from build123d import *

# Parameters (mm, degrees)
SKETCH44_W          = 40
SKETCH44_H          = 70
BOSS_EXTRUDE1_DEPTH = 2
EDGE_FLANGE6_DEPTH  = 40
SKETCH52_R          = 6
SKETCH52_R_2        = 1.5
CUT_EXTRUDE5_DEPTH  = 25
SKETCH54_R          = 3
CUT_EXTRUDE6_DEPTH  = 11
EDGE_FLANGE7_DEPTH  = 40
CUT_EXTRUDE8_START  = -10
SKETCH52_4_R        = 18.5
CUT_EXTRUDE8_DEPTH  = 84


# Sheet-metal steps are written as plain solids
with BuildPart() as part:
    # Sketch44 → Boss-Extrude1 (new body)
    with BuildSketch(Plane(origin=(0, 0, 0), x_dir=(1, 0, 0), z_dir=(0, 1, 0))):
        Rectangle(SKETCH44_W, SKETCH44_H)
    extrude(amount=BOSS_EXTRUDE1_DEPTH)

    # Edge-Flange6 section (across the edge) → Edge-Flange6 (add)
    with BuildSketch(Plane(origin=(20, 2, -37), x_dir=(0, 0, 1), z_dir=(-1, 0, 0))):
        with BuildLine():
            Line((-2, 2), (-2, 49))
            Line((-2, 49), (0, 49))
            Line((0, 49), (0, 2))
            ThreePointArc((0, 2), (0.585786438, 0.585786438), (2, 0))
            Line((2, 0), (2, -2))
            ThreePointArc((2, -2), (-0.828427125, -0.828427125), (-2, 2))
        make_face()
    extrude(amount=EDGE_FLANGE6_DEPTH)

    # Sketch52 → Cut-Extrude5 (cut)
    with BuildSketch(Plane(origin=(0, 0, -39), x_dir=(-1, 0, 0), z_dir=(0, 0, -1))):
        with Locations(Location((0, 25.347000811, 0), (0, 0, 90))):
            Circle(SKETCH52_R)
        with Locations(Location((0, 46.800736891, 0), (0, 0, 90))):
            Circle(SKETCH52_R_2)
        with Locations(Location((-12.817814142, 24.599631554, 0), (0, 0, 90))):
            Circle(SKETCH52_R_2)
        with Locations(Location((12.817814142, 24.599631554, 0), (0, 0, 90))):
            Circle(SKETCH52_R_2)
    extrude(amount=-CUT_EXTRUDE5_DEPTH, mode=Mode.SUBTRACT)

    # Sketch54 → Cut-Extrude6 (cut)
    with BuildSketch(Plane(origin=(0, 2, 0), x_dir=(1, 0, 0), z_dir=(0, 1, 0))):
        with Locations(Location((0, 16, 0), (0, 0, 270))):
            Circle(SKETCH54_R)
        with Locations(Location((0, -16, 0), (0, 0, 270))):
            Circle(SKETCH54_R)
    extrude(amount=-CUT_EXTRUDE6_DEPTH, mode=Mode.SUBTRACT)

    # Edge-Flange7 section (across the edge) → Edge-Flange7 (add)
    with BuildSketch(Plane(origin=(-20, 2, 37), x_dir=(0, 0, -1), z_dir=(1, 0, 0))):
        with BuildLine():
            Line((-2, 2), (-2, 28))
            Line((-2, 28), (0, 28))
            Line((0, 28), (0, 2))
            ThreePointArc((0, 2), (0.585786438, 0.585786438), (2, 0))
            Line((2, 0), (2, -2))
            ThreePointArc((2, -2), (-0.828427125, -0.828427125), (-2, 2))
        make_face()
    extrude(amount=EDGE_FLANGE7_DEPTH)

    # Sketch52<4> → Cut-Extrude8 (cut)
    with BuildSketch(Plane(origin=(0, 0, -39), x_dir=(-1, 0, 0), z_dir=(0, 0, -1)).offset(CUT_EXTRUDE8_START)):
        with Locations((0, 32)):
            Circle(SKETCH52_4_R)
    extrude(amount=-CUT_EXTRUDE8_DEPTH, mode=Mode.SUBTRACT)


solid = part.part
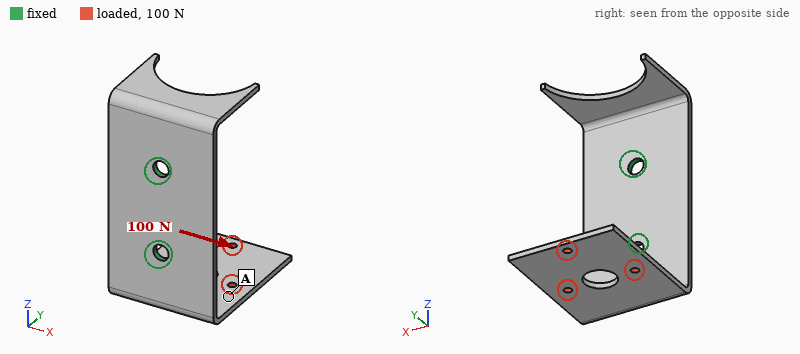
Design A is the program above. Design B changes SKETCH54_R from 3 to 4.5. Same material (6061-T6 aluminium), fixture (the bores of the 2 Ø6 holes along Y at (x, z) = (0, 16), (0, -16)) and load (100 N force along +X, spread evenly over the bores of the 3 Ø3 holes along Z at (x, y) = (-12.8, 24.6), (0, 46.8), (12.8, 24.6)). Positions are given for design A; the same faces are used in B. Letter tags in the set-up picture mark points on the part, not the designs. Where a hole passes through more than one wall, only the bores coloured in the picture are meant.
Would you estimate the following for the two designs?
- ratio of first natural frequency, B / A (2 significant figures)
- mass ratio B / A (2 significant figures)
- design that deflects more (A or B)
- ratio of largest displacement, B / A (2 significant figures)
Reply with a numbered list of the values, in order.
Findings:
1. 1.0
2. 0.99
3. A
4. 0.84
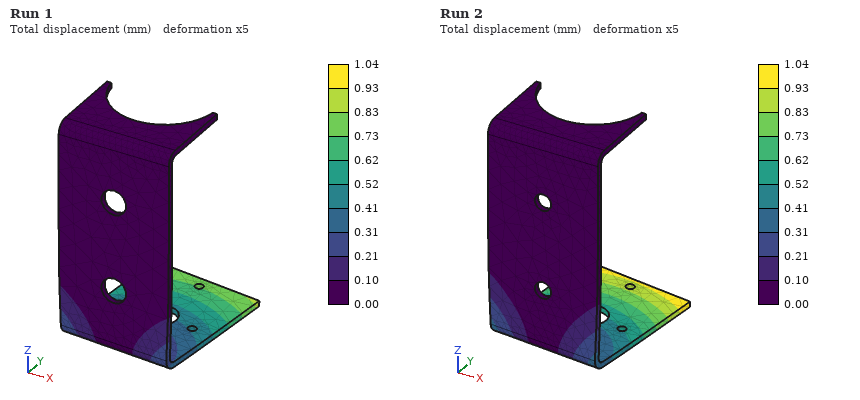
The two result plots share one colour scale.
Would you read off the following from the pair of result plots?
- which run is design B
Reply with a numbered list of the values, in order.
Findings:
1. Run 1
